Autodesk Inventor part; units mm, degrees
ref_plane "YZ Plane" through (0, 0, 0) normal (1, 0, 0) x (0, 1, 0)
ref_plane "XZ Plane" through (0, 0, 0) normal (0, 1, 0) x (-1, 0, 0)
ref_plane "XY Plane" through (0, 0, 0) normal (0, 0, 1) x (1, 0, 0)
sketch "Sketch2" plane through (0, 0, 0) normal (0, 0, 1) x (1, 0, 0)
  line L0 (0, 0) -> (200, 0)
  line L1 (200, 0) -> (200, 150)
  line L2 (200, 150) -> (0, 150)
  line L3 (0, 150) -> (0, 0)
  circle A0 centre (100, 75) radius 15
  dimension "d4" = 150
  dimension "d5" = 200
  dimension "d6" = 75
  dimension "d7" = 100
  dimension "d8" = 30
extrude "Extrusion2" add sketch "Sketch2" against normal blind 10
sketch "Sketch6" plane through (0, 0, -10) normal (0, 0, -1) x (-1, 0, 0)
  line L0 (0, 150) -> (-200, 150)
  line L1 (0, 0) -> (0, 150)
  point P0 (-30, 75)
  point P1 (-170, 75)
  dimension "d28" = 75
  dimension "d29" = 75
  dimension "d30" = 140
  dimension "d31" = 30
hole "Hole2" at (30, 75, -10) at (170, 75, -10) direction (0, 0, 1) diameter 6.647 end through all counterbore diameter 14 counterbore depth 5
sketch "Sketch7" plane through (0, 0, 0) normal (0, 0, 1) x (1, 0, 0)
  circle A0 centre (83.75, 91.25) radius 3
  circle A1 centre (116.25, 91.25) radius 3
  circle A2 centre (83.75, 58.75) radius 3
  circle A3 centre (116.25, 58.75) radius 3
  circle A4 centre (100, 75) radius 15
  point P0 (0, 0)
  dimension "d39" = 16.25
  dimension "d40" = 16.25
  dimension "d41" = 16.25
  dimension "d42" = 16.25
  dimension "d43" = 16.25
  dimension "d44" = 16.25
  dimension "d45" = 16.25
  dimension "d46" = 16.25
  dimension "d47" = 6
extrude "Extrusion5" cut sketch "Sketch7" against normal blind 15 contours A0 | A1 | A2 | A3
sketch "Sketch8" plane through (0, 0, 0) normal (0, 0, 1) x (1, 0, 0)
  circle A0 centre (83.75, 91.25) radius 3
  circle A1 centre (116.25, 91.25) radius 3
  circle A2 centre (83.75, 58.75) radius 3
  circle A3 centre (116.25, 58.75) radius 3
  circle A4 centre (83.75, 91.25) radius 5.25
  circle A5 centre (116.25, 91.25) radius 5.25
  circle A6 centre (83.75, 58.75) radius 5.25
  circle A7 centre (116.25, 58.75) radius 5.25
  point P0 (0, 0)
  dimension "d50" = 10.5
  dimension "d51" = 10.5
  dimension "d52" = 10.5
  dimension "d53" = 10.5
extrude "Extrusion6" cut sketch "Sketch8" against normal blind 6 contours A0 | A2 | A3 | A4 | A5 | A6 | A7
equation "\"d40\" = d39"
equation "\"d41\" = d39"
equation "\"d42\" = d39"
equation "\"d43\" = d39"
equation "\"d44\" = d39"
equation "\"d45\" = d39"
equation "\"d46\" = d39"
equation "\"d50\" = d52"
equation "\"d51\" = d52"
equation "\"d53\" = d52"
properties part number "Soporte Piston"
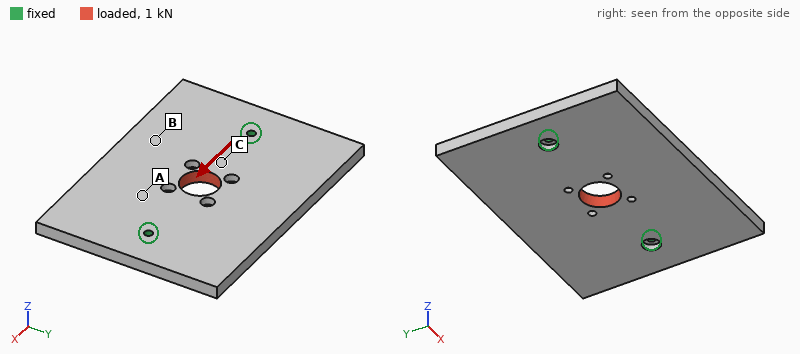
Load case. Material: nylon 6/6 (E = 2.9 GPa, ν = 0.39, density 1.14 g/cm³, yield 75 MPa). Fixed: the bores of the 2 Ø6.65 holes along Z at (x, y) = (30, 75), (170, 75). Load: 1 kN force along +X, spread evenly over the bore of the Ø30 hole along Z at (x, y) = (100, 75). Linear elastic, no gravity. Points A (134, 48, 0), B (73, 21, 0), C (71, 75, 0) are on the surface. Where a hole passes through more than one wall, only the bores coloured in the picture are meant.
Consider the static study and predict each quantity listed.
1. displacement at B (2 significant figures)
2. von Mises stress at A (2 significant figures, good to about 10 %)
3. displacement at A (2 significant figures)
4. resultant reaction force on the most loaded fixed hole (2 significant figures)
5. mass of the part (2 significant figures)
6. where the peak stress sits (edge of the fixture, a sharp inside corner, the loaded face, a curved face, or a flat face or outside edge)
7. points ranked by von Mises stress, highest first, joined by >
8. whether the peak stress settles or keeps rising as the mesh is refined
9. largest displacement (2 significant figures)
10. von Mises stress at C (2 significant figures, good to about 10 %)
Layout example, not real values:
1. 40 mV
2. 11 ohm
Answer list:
1. 24 µm
2. 0.66 MPa
3. 25 µm
4. 500 N
5. 330 g
6. edge of the fixture
7. C > A > B
8. keeps rising
9. 42 µm
10. 1.3 MPa
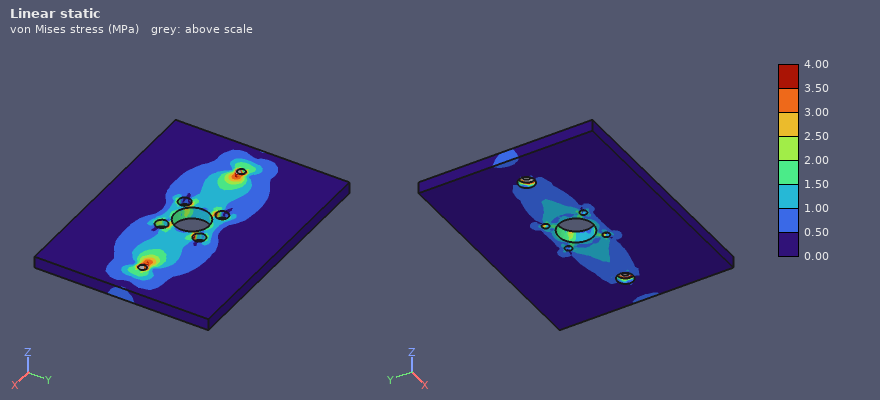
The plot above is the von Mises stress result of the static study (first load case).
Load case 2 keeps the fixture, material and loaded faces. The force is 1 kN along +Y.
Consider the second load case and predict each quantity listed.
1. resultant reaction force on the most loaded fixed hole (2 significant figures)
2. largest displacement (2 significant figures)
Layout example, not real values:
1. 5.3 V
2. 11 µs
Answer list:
1. 500 N
2. 0.26 mm
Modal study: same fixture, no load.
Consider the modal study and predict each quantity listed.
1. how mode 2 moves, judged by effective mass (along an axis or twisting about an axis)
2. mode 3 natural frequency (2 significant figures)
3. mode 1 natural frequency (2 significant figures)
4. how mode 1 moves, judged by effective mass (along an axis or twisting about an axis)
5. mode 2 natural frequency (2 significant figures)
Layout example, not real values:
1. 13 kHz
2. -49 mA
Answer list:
1. along Z
2. 380 Hz
3. 170 Hz
4. twisting about X
5. 340 Hz
